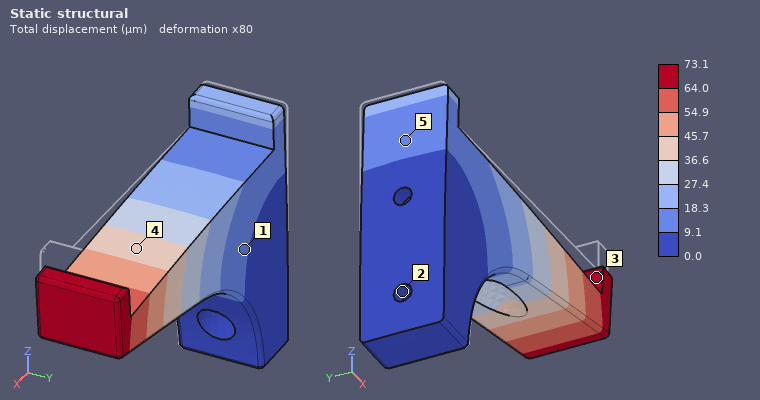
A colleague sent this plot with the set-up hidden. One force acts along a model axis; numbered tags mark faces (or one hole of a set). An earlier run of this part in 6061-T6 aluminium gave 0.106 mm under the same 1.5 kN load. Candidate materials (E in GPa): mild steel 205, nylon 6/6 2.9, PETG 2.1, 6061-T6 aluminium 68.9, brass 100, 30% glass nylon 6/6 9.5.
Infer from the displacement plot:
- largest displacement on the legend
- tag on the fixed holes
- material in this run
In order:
73.1 µm
2
brass
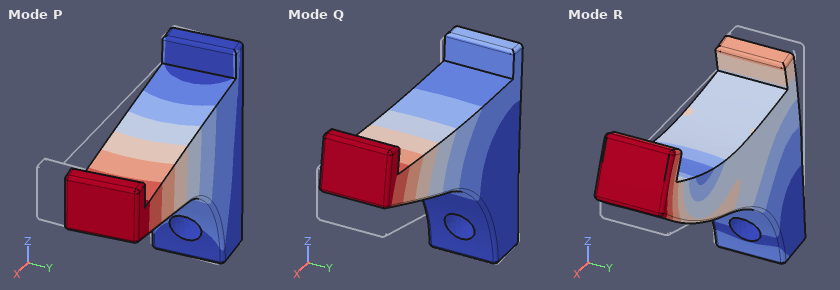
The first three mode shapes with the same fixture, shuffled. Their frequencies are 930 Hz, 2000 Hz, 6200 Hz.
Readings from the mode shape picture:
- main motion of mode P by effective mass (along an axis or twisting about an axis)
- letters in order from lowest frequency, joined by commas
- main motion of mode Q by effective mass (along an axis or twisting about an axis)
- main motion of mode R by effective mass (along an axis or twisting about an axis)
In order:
along Y
P, Q, R
along Z
along X
